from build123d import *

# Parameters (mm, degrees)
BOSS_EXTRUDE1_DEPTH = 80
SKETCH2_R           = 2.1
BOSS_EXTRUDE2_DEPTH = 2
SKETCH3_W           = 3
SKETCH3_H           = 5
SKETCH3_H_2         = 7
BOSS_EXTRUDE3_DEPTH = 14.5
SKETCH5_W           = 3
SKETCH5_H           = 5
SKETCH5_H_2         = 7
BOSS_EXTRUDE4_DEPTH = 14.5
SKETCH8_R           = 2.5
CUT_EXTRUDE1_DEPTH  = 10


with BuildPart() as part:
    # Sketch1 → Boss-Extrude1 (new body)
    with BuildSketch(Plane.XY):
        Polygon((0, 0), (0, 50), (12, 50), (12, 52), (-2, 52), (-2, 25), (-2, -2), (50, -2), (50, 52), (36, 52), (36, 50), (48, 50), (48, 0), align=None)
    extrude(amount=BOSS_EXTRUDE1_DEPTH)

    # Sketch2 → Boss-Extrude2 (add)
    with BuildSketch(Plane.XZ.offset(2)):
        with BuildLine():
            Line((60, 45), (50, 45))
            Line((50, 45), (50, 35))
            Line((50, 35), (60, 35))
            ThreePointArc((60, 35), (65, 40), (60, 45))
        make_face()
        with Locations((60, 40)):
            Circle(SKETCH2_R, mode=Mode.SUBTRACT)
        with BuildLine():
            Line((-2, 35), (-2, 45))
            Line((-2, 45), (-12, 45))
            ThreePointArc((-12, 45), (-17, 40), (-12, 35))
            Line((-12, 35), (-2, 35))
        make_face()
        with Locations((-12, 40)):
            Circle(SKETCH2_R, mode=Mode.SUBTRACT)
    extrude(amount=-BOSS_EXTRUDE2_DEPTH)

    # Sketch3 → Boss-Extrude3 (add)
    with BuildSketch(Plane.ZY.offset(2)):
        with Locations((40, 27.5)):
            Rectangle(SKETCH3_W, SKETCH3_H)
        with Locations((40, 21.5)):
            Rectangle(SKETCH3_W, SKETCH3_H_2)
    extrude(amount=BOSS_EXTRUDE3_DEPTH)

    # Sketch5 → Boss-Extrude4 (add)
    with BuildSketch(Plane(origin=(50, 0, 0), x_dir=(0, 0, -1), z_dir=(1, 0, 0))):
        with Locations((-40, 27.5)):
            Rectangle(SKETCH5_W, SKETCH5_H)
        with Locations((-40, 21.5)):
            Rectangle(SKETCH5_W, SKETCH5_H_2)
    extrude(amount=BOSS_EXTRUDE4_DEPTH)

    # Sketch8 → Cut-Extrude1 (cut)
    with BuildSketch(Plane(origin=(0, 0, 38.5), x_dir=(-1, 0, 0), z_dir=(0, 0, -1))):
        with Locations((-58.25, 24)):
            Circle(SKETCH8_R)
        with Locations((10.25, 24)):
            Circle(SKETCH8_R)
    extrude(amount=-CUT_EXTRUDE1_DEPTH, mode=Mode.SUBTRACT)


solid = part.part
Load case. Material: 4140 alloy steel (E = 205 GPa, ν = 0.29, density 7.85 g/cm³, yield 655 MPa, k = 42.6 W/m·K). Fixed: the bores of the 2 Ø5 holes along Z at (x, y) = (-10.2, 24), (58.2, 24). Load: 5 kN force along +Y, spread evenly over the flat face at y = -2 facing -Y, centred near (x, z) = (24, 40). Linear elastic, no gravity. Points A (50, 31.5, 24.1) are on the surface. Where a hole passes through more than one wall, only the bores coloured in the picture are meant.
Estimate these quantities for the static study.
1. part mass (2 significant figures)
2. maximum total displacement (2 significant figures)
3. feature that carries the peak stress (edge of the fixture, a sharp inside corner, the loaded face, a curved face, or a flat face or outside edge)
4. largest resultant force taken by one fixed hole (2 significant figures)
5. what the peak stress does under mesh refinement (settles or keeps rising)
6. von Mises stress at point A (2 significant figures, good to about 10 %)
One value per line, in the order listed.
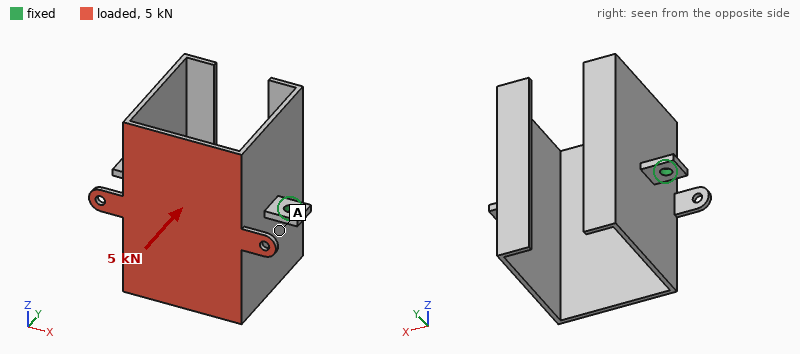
240 g
0.32 mm
edge of the fixture
2.6 kN
keeps rising
55 MPa
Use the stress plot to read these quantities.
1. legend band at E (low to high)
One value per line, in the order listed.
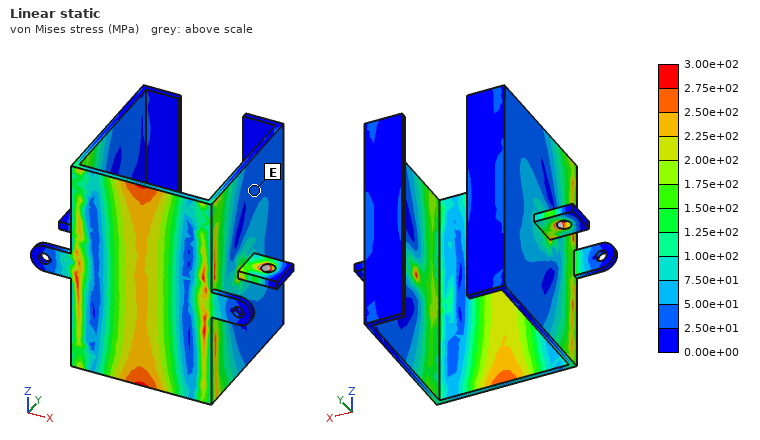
2.50e+01 to 5.00e+01 MPa
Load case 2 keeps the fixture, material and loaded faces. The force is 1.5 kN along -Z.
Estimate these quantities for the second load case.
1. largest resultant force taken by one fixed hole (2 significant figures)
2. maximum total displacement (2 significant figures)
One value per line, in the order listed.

750 N
0.67 mm
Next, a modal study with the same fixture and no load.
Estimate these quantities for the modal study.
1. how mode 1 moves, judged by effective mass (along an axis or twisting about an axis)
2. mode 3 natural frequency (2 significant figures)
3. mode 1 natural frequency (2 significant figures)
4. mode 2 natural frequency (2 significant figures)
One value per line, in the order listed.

twisting about X
830 Hz
580 Hz
620 Hz
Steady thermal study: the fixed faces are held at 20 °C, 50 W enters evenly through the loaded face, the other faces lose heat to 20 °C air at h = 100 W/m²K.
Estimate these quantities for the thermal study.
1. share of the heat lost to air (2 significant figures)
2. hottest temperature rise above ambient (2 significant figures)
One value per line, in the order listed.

94 %
59 K
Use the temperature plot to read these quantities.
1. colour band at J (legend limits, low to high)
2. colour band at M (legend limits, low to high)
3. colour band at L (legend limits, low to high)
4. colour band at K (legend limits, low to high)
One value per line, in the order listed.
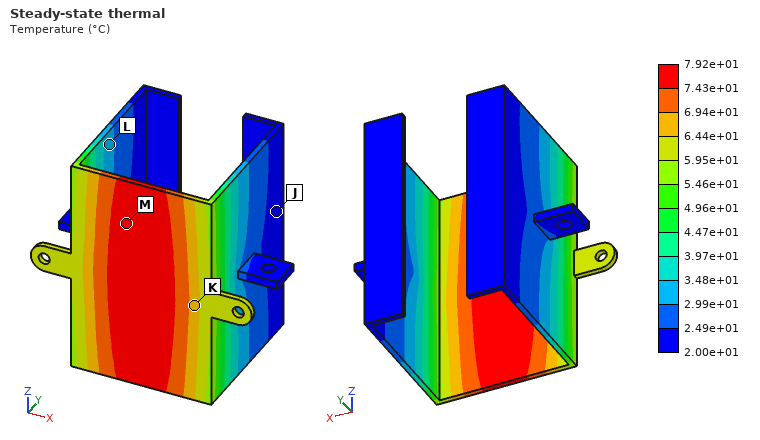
2.00e+01 to 2.49e+01 °C
7.43e+01 to 7.92e+01 °C
2.99e+01 to 3.48e+01 °C
6.44e+01 to 6.94e+01 °C
